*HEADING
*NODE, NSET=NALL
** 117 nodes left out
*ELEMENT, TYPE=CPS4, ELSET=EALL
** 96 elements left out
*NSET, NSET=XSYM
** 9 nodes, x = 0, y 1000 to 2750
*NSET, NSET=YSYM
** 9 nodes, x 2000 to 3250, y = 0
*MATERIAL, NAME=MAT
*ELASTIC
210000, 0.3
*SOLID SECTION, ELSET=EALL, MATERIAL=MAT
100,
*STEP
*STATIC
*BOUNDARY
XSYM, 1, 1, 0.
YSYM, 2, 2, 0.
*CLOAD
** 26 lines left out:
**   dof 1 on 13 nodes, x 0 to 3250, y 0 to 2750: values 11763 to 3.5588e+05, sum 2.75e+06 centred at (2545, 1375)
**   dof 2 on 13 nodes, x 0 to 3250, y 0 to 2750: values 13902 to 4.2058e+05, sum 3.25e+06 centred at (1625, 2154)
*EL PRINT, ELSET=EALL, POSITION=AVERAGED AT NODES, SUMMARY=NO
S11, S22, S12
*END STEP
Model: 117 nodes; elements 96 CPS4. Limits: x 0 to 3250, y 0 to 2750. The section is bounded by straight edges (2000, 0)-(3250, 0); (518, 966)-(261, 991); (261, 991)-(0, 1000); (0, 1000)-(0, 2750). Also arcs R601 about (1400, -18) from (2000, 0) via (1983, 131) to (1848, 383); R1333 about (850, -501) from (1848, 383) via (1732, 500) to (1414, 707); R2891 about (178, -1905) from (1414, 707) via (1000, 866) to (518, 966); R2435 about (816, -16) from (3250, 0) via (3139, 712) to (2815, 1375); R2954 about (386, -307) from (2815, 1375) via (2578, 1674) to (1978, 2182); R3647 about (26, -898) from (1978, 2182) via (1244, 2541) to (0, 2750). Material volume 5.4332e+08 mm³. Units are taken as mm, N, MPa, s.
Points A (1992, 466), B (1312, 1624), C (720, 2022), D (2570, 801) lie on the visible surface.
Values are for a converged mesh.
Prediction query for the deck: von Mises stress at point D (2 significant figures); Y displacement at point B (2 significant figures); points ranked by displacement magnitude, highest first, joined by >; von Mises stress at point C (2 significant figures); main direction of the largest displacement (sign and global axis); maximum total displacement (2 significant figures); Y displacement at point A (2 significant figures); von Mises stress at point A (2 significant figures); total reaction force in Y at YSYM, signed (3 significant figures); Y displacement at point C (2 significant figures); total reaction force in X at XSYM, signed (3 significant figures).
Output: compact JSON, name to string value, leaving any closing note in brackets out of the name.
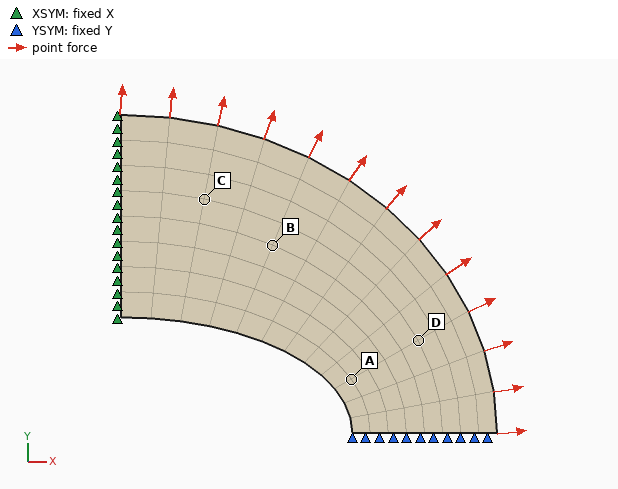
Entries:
{"von Mises stress at point D": "17 MPa", "Y displacement at point B": "0.40 mm", "points ranked by displacement magnitude, highest first, joined by >": "C > B > A > D", "von Mises stress at point C": "19 MPa", "main direction of the largest displacement": "+Y", "maximum total displacement": "0.57 mm", "Y displacement at point A": "0.13 mm", "von Mises stress at point A": "40 MPa", "total reaction force in Y at YSYM, signed": "-3.25e+06 N", "Y displacement at point C": "0.50 mm", "total reaction force in X at XSYM, signed": "-2.75e+06 N"}
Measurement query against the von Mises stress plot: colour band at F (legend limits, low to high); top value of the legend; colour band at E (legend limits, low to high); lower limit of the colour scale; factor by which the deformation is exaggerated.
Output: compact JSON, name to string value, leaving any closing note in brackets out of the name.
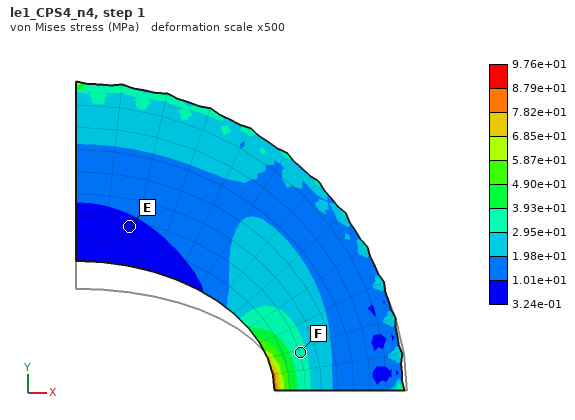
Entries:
{"colour band at F": "2.95e+01 to 3.93e+01 MPa", "top value of the legend": "9.76e+01 MPa", "colour band at E": "3.24e-01 to 1.01e+01 MPa", "lower limit of the colour scale": "3.24e-01 MPa", "factor by which the deformation is exaggerated": "500"}
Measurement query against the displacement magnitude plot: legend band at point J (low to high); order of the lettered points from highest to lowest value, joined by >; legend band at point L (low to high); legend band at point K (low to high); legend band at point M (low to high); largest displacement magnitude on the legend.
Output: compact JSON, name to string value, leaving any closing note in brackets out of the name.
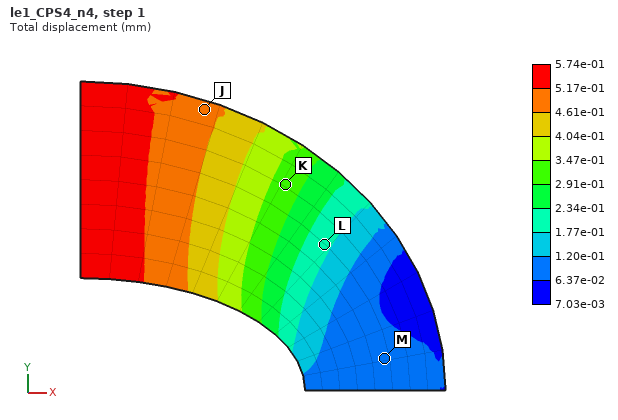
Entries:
{"legend band at point J": "4.61e-01 to 5.17e-01 mm", "order of the lettered points from highest to lowest value, joined by >": "J > K > L > M", "legend band at point L": "1.77e-01 to 2.34e-01 mm", "legend band at point K": "2.91e-01 to 3.47e-01 mm", "legend band at point M": "6.37e-02 to 1.20e-01 mm", "largest displacement magnitude on the legend": "5.74e-01 mm"}
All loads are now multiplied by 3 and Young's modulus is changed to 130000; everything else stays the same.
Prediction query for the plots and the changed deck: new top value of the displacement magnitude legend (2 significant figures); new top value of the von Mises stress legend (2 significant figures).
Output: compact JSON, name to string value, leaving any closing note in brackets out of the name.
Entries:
{"new top value of the displacement magnitude legend": "2.8 mm", "new top value of the von Mises stress legend": "290 MPa"}
